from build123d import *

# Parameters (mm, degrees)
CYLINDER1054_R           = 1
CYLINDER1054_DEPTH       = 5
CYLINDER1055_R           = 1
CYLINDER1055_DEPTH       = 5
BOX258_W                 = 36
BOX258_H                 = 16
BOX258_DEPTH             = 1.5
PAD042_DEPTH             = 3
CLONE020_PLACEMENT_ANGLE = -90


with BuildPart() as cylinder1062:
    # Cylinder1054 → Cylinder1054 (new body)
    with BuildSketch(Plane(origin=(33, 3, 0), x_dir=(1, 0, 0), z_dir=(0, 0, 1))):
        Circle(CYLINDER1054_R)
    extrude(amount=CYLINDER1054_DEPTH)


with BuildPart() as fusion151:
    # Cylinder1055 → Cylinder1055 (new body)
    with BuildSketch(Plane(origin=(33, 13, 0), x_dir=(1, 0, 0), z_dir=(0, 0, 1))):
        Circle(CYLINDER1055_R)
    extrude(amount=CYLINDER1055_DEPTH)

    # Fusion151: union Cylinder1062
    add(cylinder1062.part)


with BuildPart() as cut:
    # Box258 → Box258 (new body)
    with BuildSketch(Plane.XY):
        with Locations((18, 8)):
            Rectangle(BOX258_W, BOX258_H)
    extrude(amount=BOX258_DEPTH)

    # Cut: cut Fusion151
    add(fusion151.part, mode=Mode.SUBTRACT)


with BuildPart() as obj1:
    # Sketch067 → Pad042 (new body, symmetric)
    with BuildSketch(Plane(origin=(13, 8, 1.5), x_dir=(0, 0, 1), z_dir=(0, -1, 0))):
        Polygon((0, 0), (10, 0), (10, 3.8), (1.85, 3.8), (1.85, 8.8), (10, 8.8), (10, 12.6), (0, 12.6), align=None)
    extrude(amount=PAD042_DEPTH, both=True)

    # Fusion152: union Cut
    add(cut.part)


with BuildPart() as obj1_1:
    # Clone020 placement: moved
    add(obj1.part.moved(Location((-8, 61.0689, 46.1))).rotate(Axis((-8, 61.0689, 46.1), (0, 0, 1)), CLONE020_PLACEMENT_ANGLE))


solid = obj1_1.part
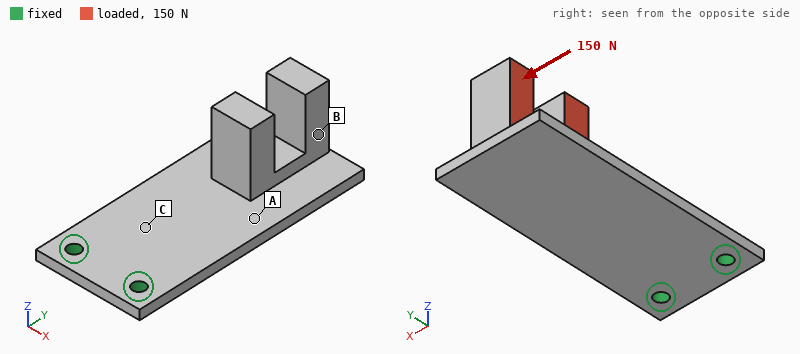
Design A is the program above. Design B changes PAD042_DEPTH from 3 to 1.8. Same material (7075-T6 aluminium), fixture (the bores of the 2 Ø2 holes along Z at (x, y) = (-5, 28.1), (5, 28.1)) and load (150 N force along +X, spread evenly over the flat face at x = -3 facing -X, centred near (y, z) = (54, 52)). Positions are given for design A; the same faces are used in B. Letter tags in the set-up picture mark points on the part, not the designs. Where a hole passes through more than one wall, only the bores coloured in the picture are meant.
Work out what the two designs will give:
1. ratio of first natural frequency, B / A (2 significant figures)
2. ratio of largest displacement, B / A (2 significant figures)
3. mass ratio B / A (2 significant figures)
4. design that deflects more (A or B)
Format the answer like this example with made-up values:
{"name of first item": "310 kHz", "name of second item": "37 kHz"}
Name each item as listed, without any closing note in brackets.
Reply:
{"ratio of first natural frequency, B / A": "1.1", "ratio of largest displacement, B / A": "1.1", "mass ratio B / A": "0.85", "design that deflects more": "B"}
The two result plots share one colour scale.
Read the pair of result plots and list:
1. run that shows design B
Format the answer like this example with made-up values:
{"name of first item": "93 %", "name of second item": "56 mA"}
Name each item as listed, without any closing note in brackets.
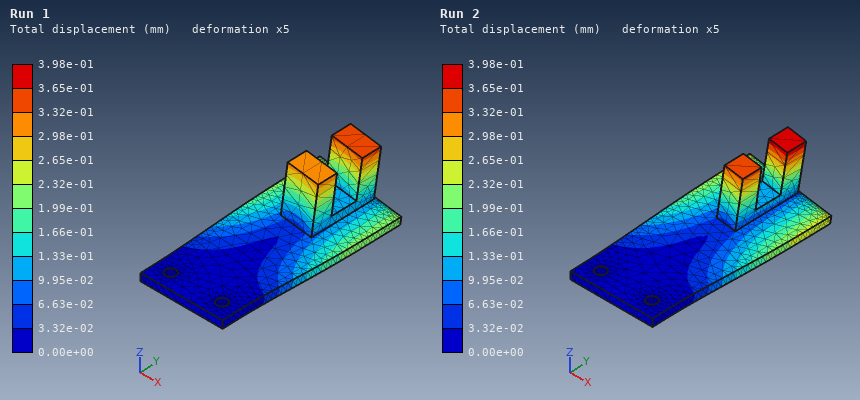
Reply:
{"run that shows design B": "Run 2"}
